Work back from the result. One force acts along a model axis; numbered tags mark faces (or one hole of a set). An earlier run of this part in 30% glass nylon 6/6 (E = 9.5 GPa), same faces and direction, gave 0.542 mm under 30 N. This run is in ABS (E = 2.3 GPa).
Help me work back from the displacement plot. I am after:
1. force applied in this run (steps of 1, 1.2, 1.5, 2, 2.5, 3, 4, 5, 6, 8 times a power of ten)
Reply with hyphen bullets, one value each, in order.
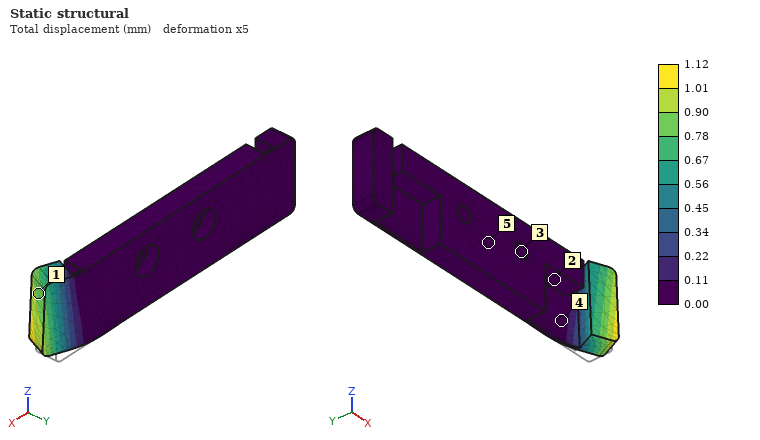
- 15 N
